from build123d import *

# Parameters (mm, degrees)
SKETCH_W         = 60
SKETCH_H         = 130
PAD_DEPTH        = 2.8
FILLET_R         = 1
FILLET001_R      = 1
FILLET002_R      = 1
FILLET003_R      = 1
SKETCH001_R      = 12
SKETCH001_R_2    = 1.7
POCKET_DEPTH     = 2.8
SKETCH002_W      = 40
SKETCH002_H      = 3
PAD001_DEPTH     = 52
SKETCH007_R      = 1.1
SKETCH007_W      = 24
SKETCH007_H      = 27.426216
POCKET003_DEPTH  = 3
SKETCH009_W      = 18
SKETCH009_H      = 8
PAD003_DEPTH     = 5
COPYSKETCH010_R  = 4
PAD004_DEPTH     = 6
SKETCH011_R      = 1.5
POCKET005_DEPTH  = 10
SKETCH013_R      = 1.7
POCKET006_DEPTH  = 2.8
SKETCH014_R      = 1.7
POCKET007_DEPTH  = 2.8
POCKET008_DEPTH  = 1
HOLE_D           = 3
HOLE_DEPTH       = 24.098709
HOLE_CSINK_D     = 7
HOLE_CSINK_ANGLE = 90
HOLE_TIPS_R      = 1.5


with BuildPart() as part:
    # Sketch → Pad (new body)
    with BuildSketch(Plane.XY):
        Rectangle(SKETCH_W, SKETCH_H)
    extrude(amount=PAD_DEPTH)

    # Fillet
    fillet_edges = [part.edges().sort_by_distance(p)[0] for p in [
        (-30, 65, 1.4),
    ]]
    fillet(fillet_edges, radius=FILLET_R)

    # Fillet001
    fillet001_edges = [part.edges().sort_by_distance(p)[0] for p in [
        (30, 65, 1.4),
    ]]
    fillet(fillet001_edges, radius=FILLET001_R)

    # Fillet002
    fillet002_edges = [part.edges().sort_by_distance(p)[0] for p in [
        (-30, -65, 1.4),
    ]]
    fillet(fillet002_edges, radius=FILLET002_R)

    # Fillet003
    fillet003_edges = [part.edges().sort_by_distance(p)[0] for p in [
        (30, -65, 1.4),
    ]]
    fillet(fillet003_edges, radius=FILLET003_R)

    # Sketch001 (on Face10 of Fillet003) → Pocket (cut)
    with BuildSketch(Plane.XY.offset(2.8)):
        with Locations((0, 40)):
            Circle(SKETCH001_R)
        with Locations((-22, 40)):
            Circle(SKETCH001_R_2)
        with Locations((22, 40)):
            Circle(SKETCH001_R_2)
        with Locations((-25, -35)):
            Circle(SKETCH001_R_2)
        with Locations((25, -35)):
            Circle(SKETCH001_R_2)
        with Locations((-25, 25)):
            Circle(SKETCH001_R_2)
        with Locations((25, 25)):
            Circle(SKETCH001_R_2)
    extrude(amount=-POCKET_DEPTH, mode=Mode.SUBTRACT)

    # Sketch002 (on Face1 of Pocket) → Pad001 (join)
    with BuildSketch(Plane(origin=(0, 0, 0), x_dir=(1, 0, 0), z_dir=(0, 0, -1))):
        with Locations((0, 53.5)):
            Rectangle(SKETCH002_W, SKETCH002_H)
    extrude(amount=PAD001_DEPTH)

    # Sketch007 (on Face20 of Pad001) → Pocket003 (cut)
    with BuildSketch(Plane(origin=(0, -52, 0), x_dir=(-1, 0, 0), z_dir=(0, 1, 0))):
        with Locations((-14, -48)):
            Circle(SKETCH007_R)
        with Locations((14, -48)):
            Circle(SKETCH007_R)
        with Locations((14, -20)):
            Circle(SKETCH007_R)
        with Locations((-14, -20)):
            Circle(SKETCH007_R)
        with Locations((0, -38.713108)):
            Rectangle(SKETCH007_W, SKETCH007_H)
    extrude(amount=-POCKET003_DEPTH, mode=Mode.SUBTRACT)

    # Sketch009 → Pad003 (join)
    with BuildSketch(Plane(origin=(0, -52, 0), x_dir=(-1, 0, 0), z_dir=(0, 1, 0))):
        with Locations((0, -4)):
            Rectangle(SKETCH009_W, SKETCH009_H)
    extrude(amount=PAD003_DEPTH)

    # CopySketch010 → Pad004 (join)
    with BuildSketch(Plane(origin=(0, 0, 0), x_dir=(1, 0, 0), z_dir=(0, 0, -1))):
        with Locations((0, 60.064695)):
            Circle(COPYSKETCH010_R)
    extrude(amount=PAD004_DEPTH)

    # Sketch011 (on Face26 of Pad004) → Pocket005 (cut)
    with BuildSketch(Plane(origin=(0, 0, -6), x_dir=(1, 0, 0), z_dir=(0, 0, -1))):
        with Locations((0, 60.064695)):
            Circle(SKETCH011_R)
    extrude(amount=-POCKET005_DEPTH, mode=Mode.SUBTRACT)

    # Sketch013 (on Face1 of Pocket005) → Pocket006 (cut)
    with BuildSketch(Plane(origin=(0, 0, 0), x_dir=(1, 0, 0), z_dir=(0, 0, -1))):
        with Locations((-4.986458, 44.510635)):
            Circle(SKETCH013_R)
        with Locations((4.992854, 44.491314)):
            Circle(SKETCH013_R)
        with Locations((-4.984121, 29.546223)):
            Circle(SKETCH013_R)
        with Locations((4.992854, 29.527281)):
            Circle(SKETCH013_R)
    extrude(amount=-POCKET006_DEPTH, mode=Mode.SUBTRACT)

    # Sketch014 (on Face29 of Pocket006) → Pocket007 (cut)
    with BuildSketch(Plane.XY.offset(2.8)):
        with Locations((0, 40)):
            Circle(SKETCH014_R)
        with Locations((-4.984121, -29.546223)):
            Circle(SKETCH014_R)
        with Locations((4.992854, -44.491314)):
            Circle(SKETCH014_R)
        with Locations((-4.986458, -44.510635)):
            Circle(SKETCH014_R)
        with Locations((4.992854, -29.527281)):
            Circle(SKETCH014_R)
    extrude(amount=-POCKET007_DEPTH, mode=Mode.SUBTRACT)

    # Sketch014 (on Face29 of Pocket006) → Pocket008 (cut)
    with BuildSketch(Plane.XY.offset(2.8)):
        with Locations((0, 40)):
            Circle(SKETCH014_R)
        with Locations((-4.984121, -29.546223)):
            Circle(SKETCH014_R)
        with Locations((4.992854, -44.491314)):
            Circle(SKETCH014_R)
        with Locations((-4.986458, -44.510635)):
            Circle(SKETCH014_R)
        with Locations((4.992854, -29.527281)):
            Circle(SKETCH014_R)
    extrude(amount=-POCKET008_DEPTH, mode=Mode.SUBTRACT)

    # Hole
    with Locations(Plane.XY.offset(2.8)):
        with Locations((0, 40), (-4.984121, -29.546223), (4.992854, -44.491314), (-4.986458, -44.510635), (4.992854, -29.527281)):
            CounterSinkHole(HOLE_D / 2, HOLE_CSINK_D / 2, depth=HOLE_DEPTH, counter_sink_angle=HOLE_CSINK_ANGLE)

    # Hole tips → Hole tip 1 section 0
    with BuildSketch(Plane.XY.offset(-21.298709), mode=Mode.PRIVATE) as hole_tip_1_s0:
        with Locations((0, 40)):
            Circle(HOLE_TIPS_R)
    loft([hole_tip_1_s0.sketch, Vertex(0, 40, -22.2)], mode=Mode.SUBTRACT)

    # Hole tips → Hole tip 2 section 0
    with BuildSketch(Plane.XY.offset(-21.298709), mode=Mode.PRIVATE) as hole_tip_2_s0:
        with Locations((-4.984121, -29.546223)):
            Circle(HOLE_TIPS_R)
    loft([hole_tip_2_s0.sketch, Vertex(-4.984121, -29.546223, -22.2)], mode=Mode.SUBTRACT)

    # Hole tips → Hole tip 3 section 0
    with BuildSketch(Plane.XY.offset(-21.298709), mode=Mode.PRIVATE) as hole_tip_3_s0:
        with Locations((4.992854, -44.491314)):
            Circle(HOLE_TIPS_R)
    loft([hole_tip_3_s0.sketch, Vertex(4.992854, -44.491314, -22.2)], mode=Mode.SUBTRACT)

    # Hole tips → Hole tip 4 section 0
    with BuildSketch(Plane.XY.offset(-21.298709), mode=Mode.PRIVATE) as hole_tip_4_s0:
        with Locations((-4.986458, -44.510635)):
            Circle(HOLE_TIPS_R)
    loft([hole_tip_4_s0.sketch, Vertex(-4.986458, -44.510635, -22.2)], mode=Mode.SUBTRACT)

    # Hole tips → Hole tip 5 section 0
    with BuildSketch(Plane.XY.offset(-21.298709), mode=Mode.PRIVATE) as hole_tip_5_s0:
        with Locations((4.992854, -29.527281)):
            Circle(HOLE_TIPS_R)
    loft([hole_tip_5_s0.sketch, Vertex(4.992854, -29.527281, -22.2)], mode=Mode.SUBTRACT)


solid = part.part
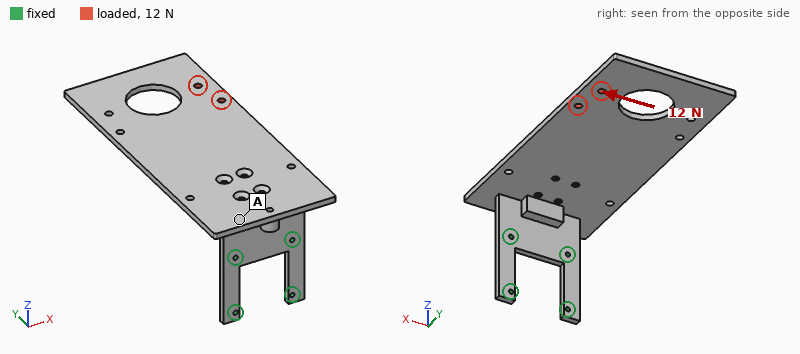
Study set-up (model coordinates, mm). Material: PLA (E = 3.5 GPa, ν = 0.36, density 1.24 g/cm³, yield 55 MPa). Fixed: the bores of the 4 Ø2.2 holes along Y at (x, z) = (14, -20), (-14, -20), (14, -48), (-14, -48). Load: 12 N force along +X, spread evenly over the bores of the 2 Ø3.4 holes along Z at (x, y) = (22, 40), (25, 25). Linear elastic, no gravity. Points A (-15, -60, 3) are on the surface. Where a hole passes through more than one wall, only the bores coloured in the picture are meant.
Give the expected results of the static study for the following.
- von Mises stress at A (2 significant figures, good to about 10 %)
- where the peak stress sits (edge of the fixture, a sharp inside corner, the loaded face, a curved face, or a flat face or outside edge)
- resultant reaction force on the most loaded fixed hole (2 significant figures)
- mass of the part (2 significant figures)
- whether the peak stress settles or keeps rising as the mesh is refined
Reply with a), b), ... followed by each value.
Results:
a) 1.5 MPa
b) edge of the fixture
c) 39 N
d) 32 g
e) keeps rising
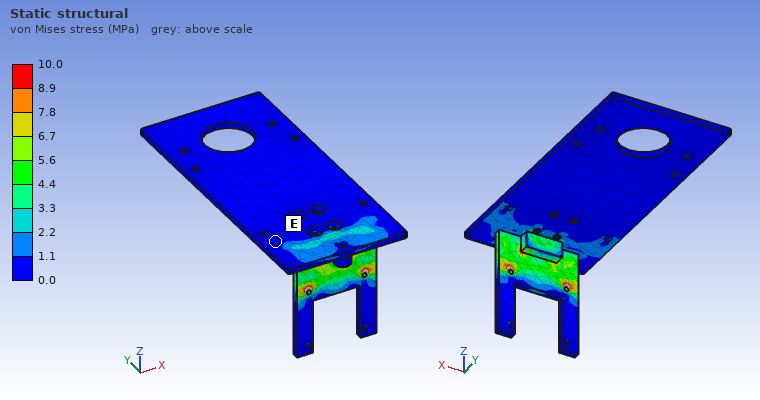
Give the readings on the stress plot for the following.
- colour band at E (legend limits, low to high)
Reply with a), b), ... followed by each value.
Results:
a) 0.0 to 1.1 MPa
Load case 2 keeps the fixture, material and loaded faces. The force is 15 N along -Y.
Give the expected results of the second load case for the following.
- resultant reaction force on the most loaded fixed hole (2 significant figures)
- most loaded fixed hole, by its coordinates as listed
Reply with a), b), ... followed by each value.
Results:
a) 21 N
b) (14, -20)
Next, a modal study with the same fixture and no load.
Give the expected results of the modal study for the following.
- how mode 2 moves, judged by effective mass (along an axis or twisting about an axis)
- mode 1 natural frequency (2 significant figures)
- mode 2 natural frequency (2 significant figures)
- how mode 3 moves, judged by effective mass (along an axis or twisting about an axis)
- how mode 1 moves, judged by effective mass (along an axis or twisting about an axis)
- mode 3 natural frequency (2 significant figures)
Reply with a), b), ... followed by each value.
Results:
a) along X
b) 45 Hz
c) 140 Hz
d) twisting about Y
e) along Z
f) 220 Hz
